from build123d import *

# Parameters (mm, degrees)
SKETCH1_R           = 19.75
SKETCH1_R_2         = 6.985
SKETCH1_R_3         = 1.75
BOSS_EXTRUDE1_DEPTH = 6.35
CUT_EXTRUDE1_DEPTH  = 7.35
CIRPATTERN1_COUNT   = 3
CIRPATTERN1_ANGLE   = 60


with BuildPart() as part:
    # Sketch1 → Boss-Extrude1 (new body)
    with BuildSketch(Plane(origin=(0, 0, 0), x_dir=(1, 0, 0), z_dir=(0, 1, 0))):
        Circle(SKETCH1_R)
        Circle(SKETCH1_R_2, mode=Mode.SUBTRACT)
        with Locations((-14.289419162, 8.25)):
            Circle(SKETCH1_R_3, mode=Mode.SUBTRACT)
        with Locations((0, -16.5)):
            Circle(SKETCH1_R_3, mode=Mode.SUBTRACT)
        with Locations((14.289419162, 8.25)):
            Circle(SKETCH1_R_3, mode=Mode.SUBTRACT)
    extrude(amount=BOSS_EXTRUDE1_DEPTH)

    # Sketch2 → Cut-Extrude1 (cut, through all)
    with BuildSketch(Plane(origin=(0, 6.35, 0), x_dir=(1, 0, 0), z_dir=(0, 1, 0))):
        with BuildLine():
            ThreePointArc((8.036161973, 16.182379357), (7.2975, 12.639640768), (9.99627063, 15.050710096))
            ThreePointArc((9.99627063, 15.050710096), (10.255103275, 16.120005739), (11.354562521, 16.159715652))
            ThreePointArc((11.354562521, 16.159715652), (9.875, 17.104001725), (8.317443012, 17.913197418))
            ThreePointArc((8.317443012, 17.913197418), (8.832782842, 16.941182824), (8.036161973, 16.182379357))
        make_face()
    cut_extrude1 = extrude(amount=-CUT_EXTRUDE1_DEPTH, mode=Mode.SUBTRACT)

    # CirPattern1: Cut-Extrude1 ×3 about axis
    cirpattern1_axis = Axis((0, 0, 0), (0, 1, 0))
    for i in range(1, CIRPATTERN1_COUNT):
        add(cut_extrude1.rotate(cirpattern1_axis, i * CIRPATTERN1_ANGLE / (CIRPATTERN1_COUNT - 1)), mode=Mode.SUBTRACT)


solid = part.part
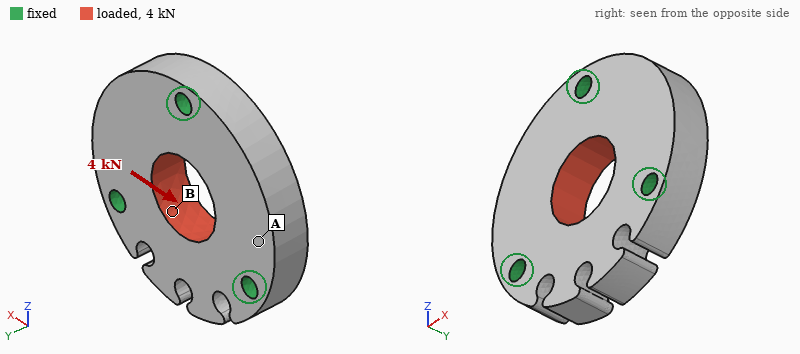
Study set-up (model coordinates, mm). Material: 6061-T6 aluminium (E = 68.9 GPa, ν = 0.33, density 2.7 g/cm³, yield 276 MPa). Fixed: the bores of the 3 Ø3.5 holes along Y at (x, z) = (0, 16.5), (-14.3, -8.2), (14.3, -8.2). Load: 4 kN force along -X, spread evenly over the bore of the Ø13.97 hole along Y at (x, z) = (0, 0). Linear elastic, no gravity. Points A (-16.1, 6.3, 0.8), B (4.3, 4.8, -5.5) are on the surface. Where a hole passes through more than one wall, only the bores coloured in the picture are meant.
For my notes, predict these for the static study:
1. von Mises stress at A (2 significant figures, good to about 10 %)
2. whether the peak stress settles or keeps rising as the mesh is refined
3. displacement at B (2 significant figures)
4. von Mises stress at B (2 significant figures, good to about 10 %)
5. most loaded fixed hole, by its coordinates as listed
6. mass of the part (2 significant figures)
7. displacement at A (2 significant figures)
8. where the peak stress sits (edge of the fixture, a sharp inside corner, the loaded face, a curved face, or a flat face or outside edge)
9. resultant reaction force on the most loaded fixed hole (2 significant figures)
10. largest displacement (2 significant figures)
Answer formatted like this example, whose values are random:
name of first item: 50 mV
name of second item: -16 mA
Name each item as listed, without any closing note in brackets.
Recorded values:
von Mises stress at A: 11 MPa
whether the peak stress settles or keeps rising as the mesh is refined: keeps rising
displacement at B: 3.1 µm
von Mises stress at B: 26 MPa
most loaded fixed hole, by its coordinates as listed: (0, 16.5)
mass of the part: 17 g
displacement at A: 3.7 µm
where the peak stress sits: edge of the fixture
resultant reaction force on the most loaded fixed hole: 1.5 kN
largest displacement: 6.1 µm
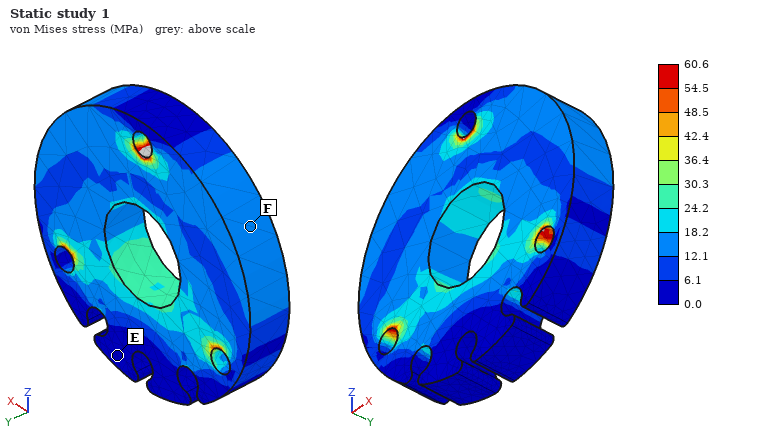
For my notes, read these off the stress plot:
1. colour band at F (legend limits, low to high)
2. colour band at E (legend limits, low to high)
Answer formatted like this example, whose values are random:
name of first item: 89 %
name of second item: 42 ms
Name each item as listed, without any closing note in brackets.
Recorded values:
colour band at F: 12.1 to 18.2 MPa
colour band at E: 0.0 to 6.1 MPa
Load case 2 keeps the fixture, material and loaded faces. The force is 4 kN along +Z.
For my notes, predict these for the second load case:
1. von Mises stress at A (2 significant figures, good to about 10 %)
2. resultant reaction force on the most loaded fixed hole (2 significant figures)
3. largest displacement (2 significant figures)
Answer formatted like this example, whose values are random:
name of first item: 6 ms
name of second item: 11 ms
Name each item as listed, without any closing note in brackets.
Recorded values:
von Mises stress at A: 12 MPa
resultant reaction force on the most loaded fixed hole: 1.4 kN
largest displacement: 9.1 µm
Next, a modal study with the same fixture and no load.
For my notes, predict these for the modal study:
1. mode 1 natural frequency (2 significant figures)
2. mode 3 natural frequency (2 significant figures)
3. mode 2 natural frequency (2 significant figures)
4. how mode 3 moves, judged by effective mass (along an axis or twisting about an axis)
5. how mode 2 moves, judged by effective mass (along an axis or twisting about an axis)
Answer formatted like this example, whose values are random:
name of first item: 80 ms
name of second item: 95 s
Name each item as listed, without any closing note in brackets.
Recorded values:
mode 1 natural frequency: 20 kHz
mode 3 natural frequency: 25 kHz
mode 2 natural frequency: 23 kHz
how mode 3 moves, judged by effective mass: along Y
how mode 2 moves, judged by effective mass: twisting about Z
